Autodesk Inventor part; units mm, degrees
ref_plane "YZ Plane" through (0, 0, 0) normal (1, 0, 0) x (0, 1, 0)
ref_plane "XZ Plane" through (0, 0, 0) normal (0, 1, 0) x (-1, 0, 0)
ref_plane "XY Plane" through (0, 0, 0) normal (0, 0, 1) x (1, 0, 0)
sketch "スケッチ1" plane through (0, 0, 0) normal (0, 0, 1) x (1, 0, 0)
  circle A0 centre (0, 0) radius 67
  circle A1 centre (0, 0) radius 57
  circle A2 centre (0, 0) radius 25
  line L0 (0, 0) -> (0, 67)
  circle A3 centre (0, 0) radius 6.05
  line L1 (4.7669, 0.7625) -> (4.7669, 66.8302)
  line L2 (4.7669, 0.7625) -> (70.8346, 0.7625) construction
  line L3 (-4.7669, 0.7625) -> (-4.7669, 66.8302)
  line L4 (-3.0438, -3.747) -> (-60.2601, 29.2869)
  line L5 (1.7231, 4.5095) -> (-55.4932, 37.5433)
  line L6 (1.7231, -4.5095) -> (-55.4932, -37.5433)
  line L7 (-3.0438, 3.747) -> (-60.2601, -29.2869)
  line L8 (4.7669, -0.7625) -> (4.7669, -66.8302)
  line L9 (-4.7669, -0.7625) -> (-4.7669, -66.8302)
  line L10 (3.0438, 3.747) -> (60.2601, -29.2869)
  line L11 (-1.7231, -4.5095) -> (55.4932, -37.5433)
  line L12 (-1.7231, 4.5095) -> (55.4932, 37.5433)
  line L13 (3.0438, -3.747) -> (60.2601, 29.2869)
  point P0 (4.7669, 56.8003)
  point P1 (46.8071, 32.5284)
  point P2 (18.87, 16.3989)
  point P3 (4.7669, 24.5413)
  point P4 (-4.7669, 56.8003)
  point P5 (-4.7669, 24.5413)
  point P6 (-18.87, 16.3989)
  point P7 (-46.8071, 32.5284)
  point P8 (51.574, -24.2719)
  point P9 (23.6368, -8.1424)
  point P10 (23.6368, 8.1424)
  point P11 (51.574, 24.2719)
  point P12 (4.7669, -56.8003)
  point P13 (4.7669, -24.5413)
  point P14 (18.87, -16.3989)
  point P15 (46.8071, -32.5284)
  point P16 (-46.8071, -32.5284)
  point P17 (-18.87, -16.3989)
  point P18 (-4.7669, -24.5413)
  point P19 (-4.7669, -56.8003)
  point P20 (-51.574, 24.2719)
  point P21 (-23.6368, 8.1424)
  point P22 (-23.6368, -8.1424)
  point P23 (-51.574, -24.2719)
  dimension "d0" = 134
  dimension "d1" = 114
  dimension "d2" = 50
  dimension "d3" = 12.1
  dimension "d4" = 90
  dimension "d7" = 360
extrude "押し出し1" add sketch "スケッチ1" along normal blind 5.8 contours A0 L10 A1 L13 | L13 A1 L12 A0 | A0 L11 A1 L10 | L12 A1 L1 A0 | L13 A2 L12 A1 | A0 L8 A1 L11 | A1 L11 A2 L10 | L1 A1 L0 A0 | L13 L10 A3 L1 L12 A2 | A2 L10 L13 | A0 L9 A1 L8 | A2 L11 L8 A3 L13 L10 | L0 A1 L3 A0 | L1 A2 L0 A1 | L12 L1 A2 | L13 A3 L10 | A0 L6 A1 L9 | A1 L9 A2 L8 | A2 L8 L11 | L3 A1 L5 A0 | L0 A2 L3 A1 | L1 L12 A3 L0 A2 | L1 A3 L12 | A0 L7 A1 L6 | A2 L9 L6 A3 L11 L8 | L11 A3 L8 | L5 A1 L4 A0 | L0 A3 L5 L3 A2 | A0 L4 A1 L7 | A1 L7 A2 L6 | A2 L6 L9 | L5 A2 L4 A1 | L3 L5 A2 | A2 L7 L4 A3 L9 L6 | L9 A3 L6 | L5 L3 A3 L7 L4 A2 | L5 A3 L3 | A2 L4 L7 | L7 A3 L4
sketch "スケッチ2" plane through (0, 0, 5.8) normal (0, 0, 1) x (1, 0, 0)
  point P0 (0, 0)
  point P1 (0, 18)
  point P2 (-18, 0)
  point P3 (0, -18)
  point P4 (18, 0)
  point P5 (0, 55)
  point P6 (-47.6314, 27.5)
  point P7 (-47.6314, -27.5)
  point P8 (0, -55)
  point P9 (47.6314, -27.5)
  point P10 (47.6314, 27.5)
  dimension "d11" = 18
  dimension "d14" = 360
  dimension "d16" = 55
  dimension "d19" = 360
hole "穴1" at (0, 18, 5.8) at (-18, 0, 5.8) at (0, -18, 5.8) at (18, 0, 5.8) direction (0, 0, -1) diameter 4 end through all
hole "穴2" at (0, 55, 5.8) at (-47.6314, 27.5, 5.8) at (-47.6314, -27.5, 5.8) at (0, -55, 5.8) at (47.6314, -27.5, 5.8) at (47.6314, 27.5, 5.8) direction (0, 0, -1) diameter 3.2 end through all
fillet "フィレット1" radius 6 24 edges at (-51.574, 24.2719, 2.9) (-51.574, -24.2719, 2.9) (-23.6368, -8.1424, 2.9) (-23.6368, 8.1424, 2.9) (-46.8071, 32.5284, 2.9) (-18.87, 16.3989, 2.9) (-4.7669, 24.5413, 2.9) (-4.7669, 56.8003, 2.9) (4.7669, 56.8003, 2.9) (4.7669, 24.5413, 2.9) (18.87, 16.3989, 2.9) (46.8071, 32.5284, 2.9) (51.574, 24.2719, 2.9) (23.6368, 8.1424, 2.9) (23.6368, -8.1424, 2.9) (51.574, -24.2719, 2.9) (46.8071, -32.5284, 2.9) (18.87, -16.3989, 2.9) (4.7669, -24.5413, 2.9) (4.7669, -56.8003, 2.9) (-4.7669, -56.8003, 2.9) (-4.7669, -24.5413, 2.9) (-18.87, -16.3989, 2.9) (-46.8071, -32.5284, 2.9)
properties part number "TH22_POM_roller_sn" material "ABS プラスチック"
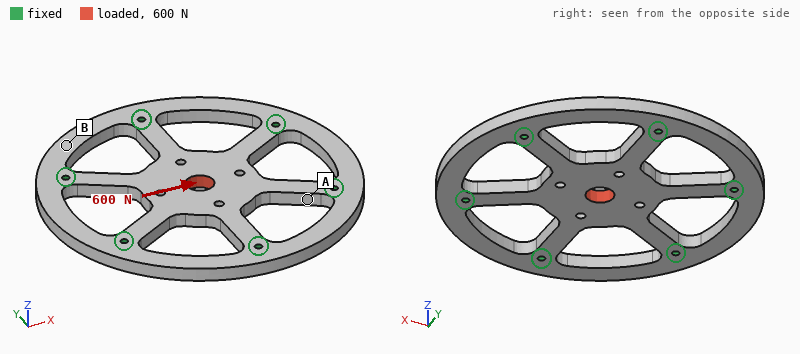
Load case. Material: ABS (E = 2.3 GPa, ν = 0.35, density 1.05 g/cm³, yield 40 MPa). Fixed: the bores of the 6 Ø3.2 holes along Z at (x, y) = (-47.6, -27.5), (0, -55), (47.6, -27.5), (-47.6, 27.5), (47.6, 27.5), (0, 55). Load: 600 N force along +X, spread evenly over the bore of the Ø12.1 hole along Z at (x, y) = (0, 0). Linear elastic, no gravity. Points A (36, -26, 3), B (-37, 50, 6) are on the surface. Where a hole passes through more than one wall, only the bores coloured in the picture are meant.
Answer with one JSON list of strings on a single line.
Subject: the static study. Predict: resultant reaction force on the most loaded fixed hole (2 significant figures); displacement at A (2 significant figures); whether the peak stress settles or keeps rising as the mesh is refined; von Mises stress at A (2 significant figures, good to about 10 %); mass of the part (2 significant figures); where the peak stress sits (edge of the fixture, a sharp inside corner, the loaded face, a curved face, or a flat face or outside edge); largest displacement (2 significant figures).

["160 N", "11 µm", "keeps rising", "2.6 MPa", "47 g", "edge of the fixture", "65 µm"]
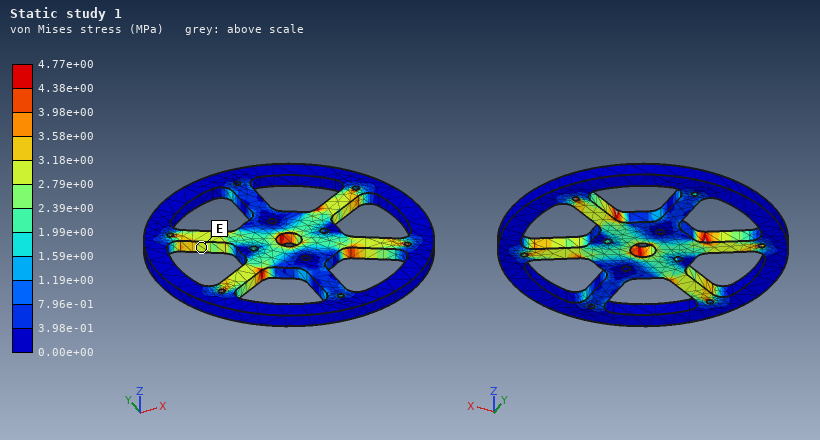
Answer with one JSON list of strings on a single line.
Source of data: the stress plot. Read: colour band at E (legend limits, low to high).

["2.79e+00 to 3.18e+00 MPa"]
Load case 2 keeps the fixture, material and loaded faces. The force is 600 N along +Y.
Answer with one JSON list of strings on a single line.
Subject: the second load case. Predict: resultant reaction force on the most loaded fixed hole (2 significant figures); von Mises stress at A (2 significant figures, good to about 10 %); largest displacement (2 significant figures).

["180 N", "2.4 MPa", "67 µm"]
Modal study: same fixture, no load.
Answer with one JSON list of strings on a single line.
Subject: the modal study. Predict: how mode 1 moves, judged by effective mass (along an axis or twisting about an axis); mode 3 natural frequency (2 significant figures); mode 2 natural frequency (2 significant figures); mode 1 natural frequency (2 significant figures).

["along Z", "1800 Hz", "1700 Hz", "870 Hz"]
